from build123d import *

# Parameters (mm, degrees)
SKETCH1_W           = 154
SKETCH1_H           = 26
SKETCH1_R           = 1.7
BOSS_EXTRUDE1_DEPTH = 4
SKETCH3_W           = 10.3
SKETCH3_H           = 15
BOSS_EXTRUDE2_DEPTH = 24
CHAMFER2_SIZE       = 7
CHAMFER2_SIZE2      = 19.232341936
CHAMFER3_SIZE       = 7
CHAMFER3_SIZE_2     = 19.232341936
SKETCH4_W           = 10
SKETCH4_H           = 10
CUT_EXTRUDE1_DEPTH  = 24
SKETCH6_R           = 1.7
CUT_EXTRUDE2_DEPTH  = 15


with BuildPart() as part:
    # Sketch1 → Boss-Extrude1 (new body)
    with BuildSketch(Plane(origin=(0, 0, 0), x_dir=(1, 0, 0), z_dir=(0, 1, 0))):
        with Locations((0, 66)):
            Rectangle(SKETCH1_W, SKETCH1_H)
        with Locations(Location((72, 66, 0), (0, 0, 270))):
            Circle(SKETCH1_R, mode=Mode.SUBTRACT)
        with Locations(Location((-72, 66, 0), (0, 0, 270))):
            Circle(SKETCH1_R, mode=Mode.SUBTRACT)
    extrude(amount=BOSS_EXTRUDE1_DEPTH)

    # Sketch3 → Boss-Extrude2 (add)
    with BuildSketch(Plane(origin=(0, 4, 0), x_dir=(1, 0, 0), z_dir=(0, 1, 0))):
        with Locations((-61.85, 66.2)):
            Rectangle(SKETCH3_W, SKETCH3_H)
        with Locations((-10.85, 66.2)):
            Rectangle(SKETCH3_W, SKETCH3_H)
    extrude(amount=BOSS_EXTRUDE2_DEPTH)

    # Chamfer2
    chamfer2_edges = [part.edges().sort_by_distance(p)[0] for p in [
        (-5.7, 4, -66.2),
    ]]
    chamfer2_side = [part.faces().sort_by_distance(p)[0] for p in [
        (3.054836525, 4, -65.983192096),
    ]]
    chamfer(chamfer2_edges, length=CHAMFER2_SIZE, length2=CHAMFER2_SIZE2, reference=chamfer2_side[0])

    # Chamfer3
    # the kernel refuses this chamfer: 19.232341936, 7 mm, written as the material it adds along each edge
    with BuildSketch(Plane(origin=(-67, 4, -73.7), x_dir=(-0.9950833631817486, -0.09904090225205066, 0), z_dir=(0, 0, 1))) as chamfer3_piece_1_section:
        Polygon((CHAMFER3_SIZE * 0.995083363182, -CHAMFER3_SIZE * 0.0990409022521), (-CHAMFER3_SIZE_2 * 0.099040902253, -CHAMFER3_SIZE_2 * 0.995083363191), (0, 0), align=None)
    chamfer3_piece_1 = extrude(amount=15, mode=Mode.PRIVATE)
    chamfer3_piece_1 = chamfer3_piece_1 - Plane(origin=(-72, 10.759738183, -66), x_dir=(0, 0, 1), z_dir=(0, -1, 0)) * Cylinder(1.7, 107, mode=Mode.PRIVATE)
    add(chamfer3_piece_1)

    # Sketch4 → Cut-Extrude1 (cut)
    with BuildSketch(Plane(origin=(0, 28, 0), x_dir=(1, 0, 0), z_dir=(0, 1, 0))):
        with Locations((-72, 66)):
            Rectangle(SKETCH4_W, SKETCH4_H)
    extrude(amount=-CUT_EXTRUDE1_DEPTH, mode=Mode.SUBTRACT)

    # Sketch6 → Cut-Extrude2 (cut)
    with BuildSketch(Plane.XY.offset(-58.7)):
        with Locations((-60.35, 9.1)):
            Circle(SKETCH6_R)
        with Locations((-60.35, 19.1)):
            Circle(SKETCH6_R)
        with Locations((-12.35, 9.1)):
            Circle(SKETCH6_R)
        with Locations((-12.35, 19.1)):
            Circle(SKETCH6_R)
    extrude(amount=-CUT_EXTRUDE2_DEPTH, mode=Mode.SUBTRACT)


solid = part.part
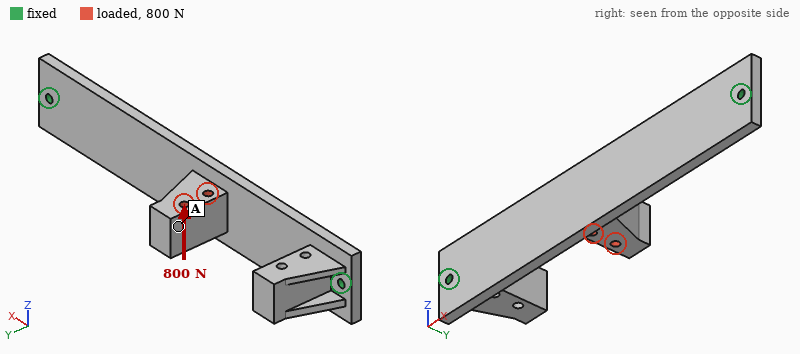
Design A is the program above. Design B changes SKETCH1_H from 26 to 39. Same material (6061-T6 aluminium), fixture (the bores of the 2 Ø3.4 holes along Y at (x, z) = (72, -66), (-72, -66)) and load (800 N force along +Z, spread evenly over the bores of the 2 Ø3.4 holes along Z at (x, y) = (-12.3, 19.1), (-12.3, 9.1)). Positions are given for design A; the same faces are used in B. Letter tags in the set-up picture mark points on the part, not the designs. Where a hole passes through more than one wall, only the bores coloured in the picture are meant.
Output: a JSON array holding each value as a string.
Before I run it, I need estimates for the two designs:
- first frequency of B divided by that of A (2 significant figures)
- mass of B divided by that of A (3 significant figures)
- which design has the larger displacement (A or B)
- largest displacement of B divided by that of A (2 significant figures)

["0.98", "1.33", "A", "0.66"]
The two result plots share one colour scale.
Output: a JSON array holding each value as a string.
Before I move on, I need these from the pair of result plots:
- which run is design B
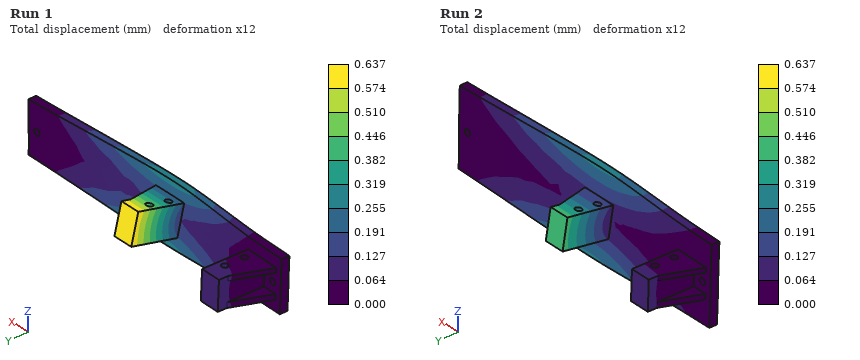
["Run 2"]
